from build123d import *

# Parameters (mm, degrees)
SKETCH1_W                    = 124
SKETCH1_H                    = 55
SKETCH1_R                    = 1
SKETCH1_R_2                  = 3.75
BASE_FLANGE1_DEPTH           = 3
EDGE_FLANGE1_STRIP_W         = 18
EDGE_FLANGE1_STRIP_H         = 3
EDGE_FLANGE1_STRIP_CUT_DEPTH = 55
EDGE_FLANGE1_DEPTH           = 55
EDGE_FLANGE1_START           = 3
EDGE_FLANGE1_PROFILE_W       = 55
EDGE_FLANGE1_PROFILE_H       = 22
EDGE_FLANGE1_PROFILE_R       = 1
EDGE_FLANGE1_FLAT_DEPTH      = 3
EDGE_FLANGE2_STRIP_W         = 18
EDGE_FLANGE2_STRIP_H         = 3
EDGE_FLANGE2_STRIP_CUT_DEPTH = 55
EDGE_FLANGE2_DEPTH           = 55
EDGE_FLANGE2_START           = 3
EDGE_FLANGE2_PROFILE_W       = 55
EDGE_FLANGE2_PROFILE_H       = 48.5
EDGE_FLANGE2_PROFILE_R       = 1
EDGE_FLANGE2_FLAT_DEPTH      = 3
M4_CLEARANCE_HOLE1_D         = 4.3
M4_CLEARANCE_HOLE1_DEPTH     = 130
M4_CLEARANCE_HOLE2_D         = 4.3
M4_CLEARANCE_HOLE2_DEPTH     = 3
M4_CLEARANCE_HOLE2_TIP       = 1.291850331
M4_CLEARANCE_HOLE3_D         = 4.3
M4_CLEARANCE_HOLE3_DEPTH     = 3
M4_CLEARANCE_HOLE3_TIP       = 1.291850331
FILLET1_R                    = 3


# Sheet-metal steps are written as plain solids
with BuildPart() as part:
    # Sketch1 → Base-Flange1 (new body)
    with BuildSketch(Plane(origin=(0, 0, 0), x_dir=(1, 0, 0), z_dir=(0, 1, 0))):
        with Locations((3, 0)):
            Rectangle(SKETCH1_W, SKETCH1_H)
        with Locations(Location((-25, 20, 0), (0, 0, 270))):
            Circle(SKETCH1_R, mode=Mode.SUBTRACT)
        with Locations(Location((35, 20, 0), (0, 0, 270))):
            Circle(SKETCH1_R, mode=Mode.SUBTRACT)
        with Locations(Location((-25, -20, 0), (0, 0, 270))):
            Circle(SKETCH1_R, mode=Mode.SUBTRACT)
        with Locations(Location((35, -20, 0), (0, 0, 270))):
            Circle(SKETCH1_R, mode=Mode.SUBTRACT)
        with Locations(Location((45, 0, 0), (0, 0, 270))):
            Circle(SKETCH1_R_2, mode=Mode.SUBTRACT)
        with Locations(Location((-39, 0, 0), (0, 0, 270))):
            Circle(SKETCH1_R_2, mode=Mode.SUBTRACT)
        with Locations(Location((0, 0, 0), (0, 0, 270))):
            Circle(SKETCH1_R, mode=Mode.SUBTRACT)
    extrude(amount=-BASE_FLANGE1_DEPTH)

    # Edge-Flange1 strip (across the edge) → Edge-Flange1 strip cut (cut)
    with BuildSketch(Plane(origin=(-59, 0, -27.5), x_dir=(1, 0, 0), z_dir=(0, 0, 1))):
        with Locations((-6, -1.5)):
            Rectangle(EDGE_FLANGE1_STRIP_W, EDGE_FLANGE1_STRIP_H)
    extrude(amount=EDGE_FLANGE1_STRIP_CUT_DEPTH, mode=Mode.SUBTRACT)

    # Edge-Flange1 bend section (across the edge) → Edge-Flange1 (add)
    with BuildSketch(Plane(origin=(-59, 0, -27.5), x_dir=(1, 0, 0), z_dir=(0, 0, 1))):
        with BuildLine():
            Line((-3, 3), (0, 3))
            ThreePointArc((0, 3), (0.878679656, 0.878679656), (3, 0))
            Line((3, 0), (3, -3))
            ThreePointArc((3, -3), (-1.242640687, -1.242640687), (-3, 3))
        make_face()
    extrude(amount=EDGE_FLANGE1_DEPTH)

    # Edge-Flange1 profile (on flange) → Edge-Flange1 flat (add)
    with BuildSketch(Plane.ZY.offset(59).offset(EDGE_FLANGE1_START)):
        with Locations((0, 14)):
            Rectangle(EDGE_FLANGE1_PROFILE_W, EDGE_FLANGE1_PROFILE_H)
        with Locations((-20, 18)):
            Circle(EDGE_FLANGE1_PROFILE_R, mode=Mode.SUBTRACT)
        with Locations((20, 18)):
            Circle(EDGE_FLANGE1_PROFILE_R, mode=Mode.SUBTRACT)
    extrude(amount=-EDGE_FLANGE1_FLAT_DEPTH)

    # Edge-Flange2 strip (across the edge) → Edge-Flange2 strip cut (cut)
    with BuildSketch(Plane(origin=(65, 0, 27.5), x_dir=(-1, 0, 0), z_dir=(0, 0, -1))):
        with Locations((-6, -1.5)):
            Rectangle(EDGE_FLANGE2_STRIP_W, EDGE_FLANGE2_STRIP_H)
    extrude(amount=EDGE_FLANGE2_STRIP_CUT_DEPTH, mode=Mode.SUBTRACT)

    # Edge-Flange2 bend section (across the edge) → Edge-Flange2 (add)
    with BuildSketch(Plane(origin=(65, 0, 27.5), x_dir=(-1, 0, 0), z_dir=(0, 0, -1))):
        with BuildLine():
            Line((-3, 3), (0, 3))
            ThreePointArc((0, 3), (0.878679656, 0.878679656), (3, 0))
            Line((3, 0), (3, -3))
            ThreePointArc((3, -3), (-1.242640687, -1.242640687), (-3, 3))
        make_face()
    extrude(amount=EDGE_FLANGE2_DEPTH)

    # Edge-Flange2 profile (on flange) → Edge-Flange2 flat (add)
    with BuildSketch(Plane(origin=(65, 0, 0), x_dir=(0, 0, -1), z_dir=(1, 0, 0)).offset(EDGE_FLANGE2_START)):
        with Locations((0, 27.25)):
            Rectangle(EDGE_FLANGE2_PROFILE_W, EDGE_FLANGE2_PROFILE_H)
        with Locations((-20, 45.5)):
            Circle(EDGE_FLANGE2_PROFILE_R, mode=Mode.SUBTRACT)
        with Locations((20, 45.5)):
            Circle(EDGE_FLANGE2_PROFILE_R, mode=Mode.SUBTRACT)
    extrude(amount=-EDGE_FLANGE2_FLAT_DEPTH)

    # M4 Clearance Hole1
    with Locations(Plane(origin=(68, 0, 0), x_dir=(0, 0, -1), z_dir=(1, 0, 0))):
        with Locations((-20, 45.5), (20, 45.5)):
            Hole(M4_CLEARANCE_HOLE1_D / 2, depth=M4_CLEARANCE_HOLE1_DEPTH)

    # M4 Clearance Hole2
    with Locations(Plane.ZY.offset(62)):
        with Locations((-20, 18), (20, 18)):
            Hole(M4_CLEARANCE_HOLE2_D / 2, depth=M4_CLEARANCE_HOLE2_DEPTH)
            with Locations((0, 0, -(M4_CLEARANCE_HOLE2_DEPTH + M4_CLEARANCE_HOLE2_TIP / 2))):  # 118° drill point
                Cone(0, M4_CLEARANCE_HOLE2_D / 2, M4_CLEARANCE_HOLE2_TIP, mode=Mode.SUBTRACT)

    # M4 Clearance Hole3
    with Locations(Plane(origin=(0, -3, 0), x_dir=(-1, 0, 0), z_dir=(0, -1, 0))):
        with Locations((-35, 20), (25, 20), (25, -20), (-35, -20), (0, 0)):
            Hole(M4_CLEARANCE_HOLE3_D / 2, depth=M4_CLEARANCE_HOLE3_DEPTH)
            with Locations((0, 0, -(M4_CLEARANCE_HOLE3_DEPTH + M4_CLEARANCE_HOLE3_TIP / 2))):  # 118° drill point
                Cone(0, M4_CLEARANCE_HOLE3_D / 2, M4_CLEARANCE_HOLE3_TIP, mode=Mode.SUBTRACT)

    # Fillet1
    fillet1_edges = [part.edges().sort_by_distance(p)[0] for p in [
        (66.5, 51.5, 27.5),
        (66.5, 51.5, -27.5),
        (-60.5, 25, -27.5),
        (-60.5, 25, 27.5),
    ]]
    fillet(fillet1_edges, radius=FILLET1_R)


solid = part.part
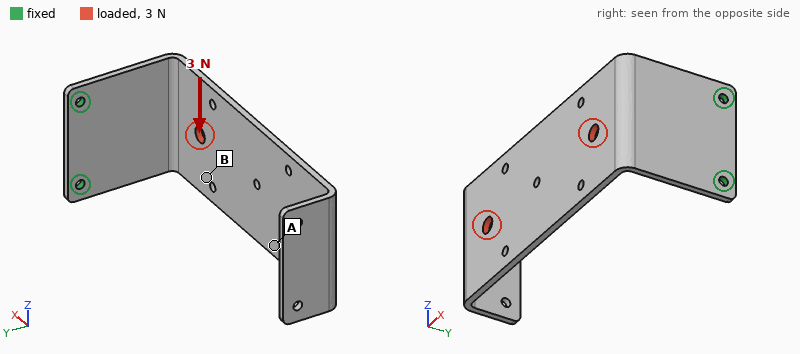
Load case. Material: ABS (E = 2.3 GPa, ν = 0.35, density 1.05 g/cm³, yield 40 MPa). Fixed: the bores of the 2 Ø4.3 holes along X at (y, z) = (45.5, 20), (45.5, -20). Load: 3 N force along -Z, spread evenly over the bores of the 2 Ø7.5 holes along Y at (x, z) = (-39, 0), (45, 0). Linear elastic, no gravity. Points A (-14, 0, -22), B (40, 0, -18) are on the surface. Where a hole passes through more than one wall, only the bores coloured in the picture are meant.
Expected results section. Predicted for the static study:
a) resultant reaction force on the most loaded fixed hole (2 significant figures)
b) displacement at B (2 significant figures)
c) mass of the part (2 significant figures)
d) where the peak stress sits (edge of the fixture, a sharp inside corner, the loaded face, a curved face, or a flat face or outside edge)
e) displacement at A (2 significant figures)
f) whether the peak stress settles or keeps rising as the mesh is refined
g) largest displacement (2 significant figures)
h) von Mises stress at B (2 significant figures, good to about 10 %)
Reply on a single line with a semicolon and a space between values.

5.9 N; 0.41 mm; 34 g; edge of the fixture; 1.1 mm; keeps rising; 1.7 mm; 0.32 MPa
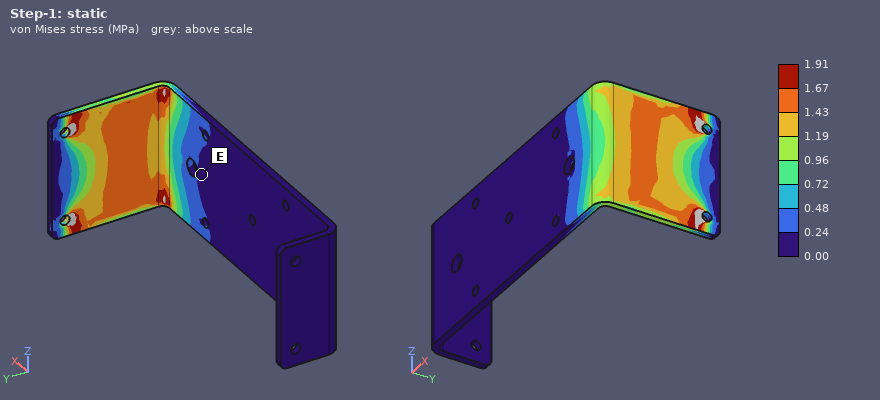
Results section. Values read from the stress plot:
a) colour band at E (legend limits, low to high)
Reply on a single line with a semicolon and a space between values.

0.00 to 0.24 MPa
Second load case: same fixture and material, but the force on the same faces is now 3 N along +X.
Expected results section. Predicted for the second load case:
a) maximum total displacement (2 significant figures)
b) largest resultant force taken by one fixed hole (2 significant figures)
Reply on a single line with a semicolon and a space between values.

1.6 mm; 1.5 N
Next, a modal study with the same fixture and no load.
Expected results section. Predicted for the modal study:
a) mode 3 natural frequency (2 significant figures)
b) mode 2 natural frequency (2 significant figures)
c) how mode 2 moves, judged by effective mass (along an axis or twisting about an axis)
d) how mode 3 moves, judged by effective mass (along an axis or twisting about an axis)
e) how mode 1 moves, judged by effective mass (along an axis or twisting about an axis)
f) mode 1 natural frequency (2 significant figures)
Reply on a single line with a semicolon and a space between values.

100 Hz; 44 Hz; along Z; along X; along Y; 22 Hz
